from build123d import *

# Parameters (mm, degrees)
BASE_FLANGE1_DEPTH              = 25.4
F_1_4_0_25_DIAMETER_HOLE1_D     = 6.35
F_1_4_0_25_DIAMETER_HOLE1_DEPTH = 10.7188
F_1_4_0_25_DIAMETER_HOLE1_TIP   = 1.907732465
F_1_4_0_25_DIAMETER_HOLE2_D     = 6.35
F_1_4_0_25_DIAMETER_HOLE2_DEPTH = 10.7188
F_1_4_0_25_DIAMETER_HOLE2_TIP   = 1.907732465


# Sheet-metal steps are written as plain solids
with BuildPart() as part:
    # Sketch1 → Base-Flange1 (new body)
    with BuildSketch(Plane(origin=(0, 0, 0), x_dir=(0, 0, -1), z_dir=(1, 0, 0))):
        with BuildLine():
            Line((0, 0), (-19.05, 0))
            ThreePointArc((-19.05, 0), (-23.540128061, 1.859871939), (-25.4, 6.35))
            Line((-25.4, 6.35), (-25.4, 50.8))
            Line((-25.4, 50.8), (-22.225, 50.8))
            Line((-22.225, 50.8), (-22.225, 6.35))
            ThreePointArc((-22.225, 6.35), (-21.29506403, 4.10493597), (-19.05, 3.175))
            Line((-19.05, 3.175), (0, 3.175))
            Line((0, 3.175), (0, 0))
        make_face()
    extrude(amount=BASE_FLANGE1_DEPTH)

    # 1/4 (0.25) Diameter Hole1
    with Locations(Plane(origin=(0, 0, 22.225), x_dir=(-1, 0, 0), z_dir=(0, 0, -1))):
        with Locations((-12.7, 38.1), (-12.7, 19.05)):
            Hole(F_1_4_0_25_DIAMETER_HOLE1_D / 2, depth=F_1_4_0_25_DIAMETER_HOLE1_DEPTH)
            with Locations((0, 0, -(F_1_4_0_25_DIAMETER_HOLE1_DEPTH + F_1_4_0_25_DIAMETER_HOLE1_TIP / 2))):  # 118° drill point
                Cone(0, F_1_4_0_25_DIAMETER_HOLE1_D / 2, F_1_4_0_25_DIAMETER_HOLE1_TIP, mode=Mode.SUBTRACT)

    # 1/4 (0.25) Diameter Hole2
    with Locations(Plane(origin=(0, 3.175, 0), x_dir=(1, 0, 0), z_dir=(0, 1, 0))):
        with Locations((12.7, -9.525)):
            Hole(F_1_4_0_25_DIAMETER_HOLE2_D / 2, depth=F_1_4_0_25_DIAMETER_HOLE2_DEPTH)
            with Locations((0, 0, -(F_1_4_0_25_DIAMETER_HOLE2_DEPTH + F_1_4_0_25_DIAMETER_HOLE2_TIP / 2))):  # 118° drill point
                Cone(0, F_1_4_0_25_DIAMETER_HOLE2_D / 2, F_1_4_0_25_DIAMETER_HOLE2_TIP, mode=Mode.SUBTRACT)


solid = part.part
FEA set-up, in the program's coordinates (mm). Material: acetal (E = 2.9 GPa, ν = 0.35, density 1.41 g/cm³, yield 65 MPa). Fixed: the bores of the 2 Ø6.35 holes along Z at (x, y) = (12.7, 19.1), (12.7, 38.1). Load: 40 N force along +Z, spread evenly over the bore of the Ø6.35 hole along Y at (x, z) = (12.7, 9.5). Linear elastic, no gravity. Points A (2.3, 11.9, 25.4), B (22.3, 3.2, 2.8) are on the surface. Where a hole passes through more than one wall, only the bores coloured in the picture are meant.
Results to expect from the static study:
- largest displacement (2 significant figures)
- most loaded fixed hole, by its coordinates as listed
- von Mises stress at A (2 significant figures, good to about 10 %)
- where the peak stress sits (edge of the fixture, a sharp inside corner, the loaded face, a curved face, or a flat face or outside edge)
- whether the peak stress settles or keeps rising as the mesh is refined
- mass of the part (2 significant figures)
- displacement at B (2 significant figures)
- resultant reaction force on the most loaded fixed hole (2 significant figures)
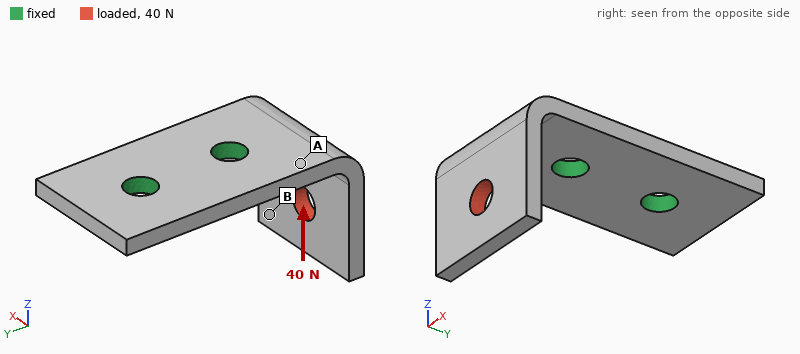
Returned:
0.69 mm
(12.7, 19.1)
7.6 MPa
edge of the fixture
keeps rising
7.6 g
0.59 mm
45 N
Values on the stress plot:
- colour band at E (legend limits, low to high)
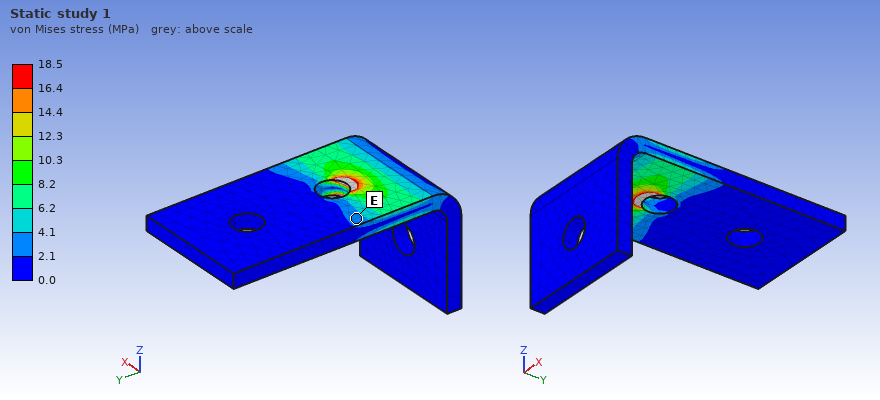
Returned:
2.1 to 4.1 MPa
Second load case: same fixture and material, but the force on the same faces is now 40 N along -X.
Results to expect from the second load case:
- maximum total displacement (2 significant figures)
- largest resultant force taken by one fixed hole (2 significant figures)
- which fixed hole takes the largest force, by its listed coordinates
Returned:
0.68 mm
60 N
(12.7, 19.1)
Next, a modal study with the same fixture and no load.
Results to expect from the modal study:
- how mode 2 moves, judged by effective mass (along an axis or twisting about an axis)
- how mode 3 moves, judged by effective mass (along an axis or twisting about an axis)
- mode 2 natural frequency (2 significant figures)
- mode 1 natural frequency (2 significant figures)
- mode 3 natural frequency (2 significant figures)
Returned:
along X
along Z
940 Hz
650 Hz
1900 Hz
